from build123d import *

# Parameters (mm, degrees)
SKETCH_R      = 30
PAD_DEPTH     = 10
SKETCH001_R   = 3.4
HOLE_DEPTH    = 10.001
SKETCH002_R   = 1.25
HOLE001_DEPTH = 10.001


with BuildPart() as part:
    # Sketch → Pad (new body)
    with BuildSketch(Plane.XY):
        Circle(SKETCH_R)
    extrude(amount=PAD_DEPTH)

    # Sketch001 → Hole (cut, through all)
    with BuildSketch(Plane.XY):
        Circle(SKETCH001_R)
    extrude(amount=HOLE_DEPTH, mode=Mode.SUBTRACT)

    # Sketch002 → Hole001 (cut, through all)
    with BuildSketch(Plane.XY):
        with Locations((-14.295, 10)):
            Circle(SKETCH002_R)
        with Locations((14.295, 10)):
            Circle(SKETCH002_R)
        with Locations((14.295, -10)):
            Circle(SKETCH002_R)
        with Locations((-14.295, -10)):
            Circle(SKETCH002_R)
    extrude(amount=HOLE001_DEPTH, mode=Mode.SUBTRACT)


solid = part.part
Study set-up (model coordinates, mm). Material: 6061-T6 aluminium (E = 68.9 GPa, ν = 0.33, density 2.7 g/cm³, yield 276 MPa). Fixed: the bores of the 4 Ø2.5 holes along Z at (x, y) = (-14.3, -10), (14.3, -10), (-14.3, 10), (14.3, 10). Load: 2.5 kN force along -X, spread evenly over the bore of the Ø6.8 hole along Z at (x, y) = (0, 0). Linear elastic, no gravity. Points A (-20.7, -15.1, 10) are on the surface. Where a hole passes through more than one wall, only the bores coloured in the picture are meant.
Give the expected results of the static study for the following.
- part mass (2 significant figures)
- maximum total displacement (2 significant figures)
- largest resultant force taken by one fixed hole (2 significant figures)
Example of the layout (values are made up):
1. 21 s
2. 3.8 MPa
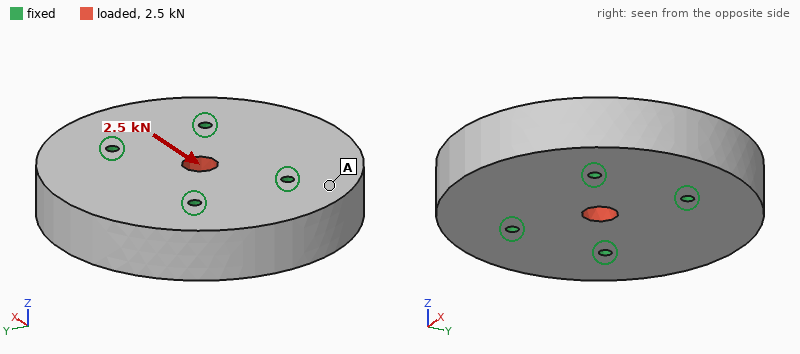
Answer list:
1. 75 g
2. 1.9 µm
3. 650 N
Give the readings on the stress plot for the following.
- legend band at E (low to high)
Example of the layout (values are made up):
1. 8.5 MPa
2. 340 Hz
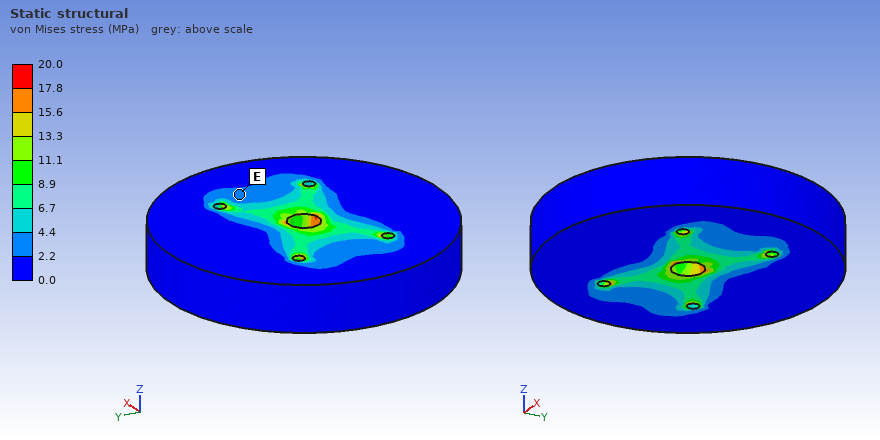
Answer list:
1. 2.2 to 4.4 MPa
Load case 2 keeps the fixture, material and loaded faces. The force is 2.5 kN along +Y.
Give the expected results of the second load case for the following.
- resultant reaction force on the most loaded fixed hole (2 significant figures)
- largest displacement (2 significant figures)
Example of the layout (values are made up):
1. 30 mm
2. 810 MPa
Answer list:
1. 650 N
2. 2.3 µm
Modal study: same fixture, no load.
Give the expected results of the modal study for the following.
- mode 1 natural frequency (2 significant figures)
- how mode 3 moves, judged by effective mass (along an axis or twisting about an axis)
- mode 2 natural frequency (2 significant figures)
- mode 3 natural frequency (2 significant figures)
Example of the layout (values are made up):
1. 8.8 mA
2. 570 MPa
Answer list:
1. 16 kHz
2. twisting about Y
3. 16 kHz
4. 25 kHz
